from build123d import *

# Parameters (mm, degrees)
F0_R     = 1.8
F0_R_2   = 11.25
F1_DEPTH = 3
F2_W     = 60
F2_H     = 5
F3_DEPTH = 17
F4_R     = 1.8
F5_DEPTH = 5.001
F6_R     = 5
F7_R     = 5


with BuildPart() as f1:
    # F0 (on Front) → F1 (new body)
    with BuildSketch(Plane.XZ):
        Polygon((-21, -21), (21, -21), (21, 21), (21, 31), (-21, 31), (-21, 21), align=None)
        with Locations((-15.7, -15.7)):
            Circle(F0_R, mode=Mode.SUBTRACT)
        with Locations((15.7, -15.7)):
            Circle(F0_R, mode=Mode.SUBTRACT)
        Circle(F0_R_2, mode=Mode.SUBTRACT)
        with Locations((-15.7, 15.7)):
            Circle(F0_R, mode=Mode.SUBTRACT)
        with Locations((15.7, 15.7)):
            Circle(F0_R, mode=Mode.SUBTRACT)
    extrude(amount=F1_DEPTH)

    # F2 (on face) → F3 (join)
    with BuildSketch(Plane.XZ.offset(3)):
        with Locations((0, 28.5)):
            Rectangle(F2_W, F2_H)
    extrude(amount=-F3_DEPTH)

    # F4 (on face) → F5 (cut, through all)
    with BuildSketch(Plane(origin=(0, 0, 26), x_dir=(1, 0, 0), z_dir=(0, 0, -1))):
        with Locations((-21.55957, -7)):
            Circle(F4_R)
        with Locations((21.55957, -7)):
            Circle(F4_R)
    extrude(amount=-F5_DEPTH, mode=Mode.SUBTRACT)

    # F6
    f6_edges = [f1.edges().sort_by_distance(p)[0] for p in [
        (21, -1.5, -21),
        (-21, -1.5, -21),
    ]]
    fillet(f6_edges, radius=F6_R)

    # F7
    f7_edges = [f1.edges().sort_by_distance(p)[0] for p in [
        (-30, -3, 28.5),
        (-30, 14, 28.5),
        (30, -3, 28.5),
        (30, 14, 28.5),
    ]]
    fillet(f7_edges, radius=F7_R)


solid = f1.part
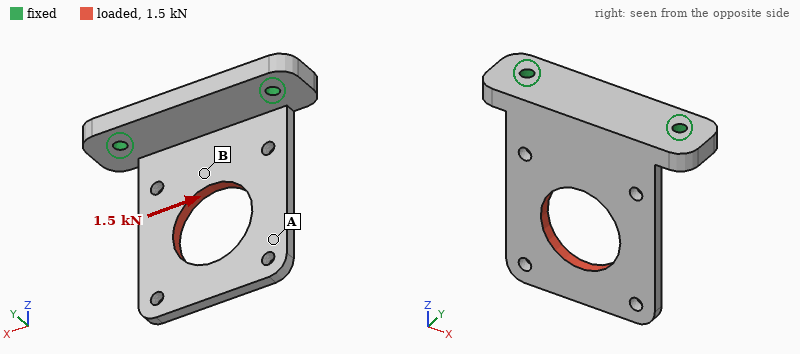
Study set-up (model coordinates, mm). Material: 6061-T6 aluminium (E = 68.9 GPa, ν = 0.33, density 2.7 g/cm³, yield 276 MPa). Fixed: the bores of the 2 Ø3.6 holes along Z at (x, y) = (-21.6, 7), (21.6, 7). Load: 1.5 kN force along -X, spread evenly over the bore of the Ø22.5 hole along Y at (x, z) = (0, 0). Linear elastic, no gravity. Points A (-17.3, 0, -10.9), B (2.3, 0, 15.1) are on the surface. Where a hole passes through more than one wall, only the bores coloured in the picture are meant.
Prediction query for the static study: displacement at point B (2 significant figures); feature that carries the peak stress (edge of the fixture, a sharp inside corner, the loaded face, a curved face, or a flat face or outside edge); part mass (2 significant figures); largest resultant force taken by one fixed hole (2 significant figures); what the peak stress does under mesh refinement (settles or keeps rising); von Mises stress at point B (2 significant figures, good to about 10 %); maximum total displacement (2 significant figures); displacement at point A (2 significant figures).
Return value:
0.029 mm
edge of the fixture
26 g
1.3 kN
keeps rising
54 MPa
0.14 mm
0.12 mm
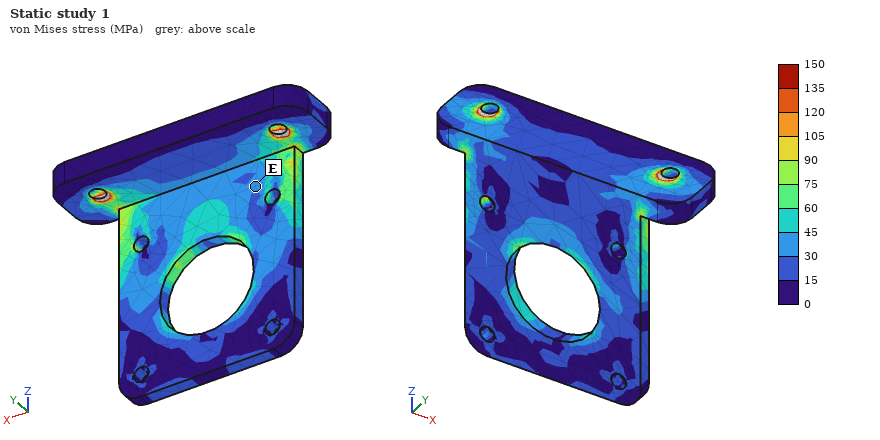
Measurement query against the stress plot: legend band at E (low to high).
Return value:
30 to 45 MPa
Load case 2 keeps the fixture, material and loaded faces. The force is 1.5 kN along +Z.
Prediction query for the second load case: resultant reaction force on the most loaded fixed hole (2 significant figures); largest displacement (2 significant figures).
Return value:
760 N
0.14 mm
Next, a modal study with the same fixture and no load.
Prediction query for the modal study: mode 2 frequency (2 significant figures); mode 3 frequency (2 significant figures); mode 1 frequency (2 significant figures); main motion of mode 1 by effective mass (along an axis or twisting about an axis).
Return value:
2500 Hz
5500 Hz
990 Hz
along Y
